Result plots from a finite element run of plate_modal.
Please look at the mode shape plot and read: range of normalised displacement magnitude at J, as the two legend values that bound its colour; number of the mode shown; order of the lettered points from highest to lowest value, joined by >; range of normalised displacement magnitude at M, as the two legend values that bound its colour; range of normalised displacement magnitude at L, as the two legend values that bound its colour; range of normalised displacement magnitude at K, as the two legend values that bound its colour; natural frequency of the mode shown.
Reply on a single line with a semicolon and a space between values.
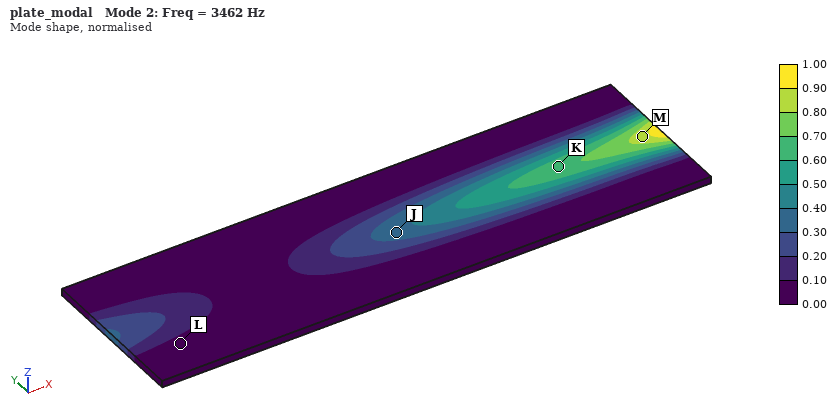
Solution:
0.30 to 0.40; 2; M > K > J > L; 0.80 to 0.90; 0.00 to 0.10; 0.60 to 0.70; 3462 Hz
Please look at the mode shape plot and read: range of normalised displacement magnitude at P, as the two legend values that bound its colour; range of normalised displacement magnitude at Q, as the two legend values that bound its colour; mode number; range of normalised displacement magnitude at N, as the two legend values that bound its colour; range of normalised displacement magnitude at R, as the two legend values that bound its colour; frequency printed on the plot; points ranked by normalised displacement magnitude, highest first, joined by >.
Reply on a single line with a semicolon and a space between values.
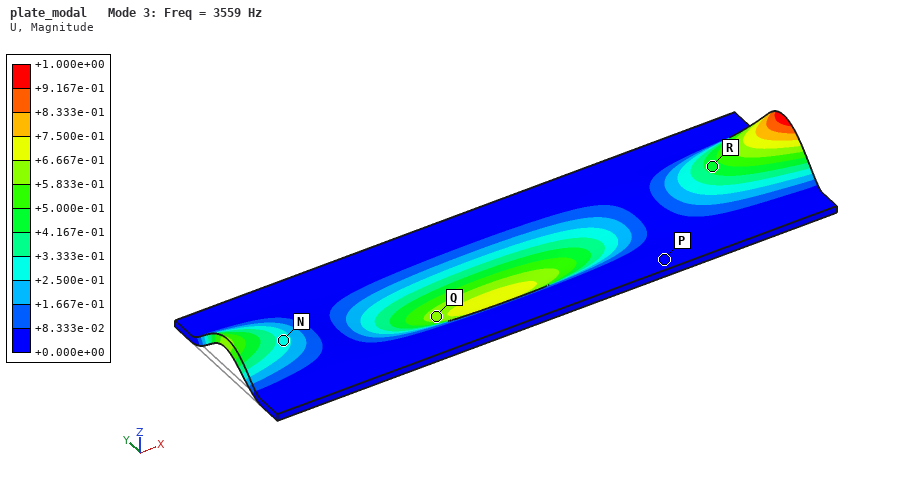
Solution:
+0.000e+00 to +8.333e-02; +5.833e-01 to +6.667e-01; 3; +2.500e-01 to +3.333e-01; +4.167e-01 to +5.000e-01; 3559 Hz; Q > R > N > P
